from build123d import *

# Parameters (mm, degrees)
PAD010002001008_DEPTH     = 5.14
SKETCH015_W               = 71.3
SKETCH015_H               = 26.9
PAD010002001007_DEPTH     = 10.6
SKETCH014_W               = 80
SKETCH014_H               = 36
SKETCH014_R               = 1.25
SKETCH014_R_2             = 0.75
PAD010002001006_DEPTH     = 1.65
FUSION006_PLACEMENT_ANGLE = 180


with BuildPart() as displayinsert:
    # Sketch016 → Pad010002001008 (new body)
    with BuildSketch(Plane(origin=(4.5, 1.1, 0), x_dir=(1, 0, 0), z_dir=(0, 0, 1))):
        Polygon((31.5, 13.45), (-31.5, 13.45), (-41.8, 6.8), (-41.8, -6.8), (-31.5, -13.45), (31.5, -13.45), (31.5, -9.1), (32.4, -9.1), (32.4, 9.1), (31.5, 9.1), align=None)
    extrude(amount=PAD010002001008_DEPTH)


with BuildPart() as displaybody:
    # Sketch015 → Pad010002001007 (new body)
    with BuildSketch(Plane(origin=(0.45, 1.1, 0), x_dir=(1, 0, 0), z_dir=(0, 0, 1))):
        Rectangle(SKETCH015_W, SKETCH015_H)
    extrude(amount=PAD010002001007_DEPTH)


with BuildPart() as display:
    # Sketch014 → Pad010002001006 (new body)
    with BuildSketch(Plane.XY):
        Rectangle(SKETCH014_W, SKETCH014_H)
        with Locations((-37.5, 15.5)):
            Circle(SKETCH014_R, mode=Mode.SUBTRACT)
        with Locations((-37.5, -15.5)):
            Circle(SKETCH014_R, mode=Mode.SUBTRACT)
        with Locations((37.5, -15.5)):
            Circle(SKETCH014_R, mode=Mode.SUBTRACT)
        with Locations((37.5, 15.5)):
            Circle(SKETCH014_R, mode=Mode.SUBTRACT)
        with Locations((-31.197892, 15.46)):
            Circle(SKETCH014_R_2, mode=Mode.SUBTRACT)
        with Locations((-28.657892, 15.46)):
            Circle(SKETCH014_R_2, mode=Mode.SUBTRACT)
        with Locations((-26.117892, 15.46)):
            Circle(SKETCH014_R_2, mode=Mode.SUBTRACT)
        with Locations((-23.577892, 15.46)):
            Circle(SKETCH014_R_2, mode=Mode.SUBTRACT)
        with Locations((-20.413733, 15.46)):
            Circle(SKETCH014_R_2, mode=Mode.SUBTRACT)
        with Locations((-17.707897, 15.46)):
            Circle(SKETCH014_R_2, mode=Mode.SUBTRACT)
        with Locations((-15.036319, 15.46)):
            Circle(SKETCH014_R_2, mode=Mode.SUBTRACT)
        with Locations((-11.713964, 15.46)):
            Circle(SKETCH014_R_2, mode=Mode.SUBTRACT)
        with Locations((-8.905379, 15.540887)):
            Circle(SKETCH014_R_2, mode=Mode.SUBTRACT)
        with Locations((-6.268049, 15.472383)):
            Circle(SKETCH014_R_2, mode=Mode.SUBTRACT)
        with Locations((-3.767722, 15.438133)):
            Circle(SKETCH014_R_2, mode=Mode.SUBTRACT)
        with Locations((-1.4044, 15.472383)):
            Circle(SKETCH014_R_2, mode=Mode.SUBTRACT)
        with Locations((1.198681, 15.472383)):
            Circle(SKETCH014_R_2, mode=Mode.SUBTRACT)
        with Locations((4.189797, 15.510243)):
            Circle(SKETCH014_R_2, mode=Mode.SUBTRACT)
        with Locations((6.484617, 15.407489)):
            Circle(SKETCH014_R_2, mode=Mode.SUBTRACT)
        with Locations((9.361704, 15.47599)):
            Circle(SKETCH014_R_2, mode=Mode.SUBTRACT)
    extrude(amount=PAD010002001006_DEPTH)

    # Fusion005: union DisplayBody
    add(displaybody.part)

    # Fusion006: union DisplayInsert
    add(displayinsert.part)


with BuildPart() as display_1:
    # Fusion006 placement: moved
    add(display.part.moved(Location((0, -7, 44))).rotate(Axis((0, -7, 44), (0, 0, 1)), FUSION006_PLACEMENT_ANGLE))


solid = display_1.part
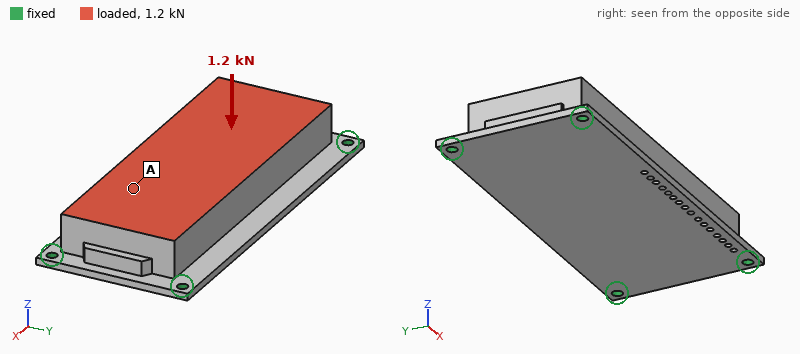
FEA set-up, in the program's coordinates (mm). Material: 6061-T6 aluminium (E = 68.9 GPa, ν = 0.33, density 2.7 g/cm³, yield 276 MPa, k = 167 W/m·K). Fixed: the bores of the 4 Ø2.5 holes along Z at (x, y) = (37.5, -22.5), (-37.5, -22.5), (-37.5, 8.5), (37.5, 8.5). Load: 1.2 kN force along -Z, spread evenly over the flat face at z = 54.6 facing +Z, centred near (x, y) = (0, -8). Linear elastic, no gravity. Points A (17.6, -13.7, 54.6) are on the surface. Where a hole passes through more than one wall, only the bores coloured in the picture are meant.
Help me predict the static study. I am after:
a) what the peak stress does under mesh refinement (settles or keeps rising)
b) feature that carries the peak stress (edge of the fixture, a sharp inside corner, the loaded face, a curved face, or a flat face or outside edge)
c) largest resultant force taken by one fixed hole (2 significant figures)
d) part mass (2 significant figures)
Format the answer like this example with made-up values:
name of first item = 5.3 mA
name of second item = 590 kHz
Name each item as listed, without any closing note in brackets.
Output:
what the peak stress does under mesh refinement = keeps rising
feature that carries the peak stress = edge of the fixture
largest resultant force taken by one fixed hole = 520 N
part mass = 59 g
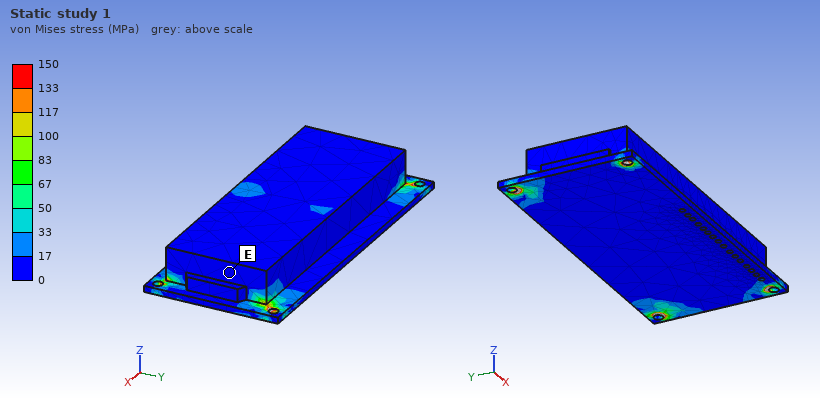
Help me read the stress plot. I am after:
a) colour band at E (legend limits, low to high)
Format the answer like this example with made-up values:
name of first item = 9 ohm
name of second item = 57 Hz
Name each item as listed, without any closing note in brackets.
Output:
colour band at E = 0 to 17 MPa
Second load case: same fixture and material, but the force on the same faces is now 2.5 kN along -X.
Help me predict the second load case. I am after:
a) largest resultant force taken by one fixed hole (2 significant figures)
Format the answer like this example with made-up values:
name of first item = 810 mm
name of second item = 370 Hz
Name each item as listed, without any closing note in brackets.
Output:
largest resultant force taken by one fixed hole = 790 N
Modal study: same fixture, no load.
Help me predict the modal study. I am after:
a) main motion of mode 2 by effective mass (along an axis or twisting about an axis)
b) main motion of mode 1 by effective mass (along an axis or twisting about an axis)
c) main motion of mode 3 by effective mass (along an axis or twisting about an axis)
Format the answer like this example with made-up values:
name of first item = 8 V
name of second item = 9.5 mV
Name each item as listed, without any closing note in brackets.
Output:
main motion of mode 2 by effective mass = along Y
main motion of mode 1 by effective mass = along Z
main motion of mode 3 by effective mass = twisting about Y
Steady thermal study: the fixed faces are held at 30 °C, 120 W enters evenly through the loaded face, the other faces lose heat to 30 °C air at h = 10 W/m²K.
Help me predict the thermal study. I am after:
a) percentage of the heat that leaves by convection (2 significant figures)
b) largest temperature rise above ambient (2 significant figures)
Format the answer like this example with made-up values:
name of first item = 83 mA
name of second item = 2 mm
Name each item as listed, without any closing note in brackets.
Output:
percentage of the heat that leaves by convection = 3.4 %
largest temperature rise above ambient = 83 K
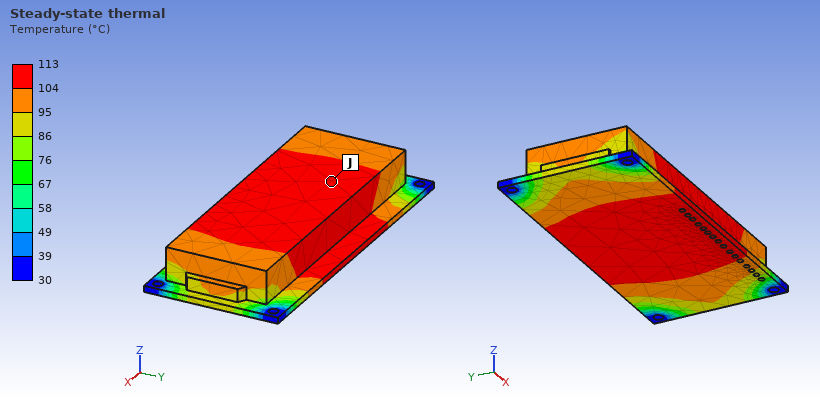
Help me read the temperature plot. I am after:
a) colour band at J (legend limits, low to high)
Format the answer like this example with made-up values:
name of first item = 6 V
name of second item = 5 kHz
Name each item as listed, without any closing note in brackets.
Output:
colour band at J = 104 to 113 °C
